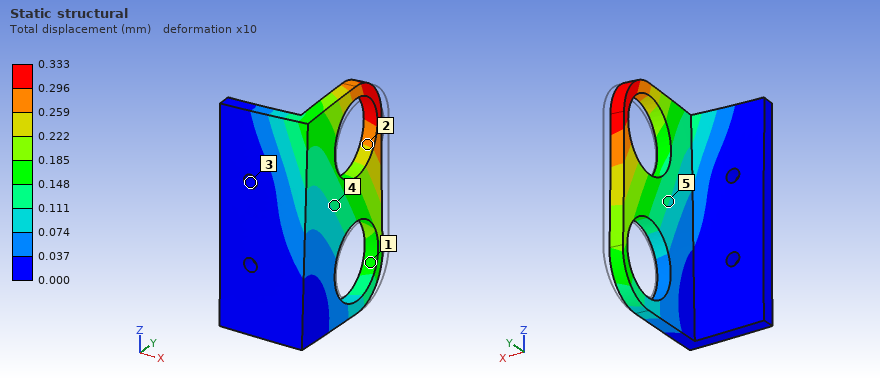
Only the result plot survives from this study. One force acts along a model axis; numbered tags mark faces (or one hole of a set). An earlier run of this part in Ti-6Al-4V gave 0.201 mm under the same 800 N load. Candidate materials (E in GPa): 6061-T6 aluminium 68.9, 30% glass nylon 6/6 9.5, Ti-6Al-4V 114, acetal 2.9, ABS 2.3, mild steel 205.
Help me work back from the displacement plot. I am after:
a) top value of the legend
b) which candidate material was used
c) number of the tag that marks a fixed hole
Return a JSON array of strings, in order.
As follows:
["0.333 mm", "6061-T6 aluminium", "3"]
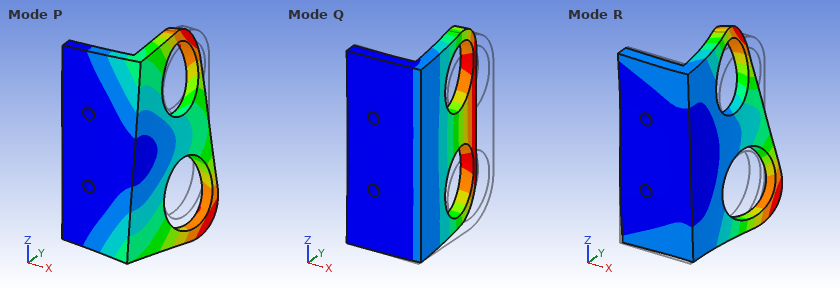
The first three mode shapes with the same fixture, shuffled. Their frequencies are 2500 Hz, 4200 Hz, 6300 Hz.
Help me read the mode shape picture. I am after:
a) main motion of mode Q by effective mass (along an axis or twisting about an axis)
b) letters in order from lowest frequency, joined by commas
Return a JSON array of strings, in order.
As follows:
["along X", "Q, P, R"]
